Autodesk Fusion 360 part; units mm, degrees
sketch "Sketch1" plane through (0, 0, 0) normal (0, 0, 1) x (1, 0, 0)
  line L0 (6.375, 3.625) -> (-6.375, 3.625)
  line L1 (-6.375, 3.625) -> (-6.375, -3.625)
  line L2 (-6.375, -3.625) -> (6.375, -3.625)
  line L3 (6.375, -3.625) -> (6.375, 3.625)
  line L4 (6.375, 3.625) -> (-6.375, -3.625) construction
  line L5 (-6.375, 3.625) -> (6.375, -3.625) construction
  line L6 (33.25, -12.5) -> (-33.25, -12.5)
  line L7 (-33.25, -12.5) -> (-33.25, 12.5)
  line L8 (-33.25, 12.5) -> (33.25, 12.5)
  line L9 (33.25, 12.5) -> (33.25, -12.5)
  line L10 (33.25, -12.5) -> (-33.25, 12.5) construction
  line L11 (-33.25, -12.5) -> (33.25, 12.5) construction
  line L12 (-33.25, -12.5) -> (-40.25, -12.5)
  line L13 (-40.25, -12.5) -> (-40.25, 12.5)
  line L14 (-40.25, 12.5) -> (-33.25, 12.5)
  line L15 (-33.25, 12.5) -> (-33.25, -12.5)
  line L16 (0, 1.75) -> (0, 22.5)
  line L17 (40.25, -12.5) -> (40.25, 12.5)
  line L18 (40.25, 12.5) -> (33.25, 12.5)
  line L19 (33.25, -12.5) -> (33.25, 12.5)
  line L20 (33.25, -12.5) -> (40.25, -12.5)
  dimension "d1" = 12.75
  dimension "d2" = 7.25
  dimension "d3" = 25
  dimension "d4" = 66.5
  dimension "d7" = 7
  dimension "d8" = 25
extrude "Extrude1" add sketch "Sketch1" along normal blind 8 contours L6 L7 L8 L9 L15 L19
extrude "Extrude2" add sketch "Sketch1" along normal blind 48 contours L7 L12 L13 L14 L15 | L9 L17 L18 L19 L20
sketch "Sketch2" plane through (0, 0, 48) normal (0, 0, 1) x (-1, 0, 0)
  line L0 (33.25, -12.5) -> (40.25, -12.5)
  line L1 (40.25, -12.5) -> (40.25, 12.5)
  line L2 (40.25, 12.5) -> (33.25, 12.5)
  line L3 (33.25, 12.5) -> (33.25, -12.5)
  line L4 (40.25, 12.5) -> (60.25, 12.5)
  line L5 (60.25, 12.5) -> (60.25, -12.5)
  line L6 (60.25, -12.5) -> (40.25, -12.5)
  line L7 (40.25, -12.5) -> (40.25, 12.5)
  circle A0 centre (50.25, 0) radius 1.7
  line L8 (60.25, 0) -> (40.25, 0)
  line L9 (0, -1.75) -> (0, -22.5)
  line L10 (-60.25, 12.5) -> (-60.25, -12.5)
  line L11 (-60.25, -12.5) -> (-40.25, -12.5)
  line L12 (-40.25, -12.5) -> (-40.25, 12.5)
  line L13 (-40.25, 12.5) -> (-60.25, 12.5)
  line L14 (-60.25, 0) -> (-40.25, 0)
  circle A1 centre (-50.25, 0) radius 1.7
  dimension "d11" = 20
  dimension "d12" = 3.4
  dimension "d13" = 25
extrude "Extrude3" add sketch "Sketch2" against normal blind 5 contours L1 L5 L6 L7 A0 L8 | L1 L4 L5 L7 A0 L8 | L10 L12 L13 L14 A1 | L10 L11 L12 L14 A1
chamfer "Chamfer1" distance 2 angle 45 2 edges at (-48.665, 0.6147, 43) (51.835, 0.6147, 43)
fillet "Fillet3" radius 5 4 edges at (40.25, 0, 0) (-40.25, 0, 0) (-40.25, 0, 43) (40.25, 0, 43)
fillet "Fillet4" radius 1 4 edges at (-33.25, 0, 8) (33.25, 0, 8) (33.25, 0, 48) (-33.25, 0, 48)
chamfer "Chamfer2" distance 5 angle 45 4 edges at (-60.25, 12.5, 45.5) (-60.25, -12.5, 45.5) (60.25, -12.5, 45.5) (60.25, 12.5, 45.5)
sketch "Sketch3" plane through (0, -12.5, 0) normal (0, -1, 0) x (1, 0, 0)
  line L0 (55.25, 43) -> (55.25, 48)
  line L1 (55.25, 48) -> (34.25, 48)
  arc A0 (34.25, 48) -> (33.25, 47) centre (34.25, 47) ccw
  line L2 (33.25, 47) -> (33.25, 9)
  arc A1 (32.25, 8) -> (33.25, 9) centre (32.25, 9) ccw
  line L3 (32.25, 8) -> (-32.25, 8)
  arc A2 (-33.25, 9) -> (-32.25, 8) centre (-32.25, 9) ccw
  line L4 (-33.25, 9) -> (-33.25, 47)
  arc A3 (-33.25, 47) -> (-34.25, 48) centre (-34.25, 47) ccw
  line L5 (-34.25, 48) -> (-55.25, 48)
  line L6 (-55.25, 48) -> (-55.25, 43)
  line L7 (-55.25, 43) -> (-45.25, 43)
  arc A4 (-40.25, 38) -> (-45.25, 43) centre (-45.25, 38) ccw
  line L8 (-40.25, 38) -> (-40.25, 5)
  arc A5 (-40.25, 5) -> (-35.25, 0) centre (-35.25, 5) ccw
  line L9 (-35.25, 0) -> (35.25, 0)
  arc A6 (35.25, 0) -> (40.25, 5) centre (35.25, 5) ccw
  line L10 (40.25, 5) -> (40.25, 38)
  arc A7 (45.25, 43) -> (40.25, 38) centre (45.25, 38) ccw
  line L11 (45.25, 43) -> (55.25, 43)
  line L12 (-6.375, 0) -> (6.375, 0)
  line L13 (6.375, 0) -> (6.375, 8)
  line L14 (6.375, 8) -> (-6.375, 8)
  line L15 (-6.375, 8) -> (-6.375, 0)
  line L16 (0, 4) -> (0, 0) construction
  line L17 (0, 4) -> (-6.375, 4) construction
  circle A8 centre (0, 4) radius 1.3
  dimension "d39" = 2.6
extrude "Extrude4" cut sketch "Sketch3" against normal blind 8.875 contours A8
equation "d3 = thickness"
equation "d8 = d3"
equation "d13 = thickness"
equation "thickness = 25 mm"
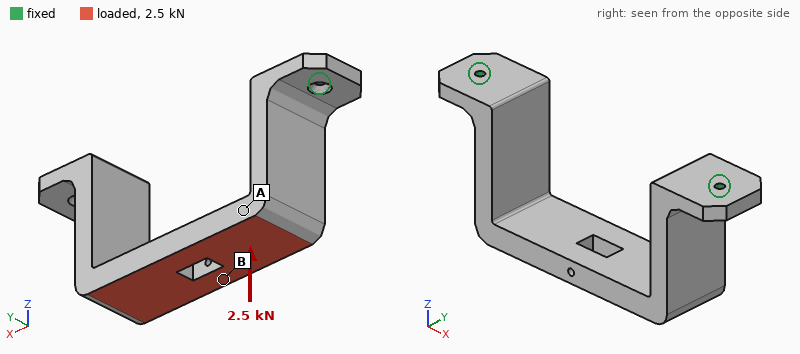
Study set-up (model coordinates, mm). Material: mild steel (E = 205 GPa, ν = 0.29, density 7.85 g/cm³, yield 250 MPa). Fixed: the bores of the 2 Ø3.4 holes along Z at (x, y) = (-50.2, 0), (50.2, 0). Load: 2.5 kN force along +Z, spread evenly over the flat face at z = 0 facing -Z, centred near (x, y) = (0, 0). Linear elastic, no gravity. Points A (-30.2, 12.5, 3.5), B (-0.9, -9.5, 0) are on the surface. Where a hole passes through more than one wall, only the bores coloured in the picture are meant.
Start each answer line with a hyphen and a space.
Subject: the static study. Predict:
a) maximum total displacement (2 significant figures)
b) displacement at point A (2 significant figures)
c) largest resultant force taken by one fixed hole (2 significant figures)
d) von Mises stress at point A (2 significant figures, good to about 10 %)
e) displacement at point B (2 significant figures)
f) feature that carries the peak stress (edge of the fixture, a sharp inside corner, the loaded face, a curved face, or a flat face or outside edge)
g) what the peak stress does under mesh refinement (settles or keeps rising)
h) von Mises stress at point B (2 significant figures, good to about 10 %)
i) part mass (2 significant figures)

- 34 µm
- 14 µm
- 1.4 kN
- 16 MPa
- 34 µm
- edge of the fixture
- keeps rising
- 53 MPa
- 270 g
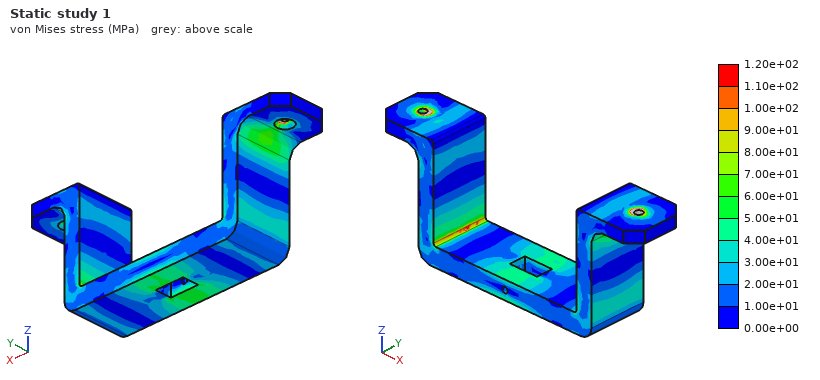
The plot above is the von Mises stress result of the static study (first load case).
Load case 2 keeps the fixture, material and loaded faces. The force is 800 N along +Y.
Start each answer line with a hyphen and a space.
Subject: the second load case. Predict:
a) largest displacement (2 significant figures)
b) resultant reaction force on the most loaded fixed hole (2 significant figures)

- 0.20 mm
- 400 N
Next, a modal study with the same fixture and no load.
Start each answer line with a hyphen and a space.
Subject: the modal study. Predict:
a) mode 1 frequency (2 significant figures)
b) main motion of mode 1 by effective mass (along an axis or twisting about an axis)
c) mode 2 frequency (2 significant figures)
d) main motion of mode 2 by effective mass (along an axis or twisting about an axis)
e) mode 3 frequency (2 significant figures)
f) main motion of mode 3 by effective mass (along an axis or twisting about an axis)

- 910 Hz
- along Y
- 1800 Hz
- along X
- 2400 Hz
- twisting about Z
